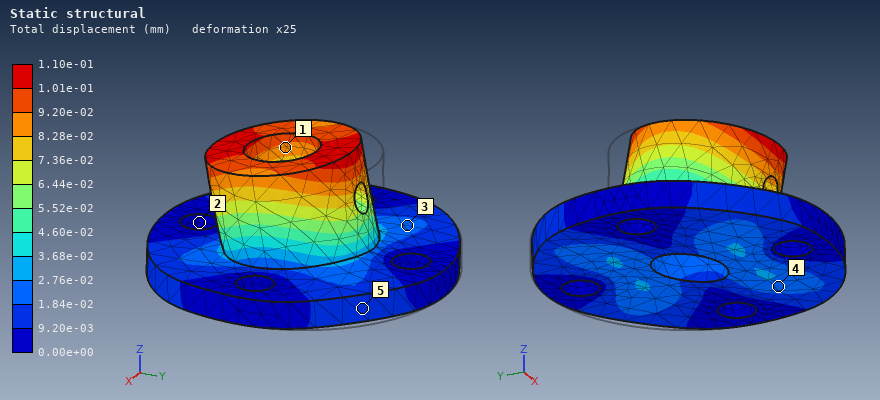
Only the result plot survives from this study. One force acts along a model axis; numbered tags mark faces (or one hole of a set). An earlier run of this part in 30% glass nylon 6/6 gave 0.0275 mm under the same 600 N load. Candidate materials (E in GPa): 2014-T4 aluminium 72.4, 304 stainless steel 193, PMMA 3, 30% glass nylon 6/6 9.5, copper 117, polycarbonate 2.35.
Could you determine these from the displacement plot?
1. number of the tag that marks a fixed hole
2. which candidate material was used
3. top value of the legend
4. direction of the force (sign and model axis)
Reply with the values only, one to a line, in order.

2
polycarbonate
1.10e-01 mm
-Y
